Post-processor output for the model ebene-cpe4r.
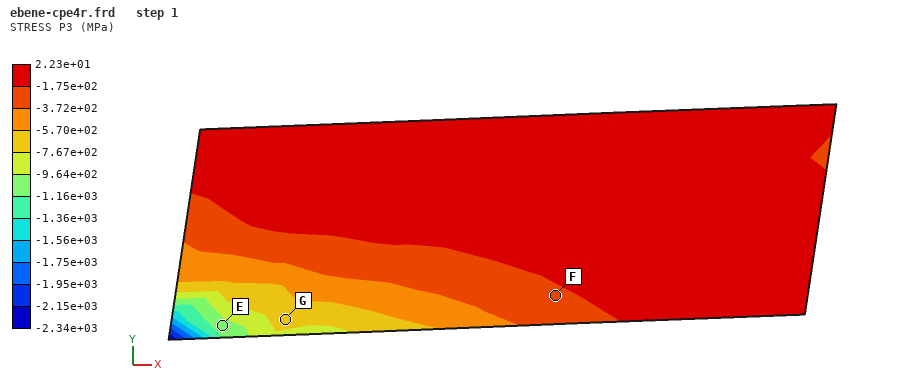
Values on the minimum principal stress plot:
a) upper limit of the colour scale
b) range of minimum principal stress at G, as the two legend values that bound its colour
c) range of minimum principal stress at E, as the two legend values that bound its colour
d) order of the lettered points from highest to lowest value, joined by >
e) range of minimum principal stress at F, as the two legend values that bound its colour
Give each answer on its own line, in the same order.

2.23e+01 MPa
-7.67e+02 to -5.70e+02 MPa
-1.16e+03 to -9.64e+02 MPa
F > G > E
-3.72e+02 to -1.75e+02 MPa
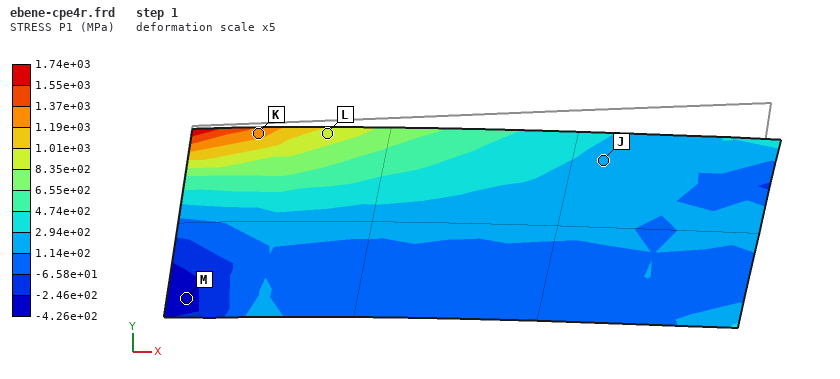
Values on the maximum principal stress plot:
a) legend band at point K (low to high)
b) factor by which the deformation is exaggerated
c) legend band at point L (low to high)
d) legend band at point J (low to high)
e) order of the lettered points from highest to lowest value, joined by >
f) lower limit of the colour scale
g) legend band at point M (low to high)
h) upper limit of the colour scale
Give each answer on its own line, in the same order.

1.19e+03 to 1.37e+03 MPa
5
8.35e+02 to 1.01e+03 MPa
1.14e+02 to 2.94e+02 MPa
K > L > J > M
-4.26e+02 MPa
-4.26e+02 to -2.46e+02 MPa
1.74e+03 MPa
